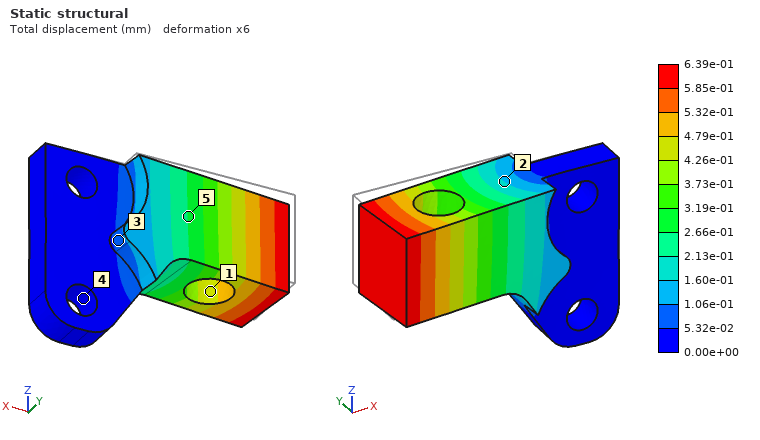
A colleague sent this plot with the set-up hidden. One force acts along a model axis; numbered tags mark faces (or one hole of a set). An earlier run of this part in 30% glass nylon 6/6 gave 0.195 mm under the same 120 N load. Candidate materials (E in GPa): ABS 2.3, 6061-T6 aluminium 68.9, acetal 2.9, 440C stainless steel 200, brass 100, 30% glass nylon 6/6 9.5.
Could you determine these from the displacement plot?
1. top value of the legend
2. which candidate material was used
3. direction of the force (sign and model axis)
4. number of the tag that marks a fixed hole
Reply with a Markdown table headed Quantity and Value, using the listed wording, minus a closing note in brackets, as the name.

| Quantity | Value |
|---|---|
| top value of the legend | 6.39e-01 mm |
| which candidate material was used | acetal |
| direction of the force | -Y |
| number of the tag that marks a fixed hole | 4 |
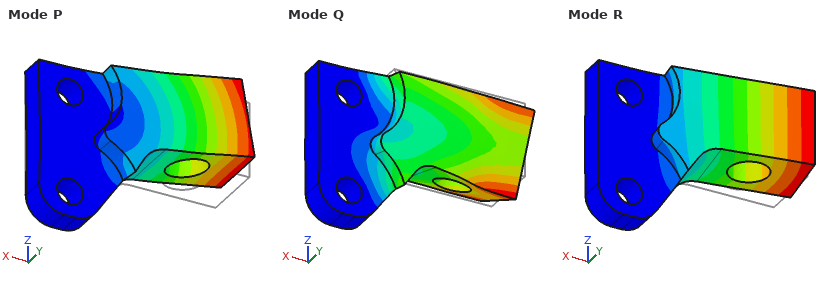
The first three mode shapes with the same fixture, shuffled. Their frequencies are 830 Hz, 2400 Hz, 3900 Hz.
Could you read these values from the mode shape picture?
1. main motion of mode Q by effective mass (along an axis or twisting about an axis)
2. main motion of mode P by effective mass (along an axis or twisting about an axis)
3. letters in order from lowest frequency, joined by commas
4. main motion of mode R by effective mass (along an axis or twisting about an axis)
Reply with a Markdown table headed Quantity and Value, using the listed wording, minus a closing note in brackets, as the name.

| Quantity | Value |
|---|---|
| main motion of mode Q by effective mass | twisting about X |
| main motion of mode P by effective mass | along Z |
| letters in order from lowest frequency, joined by commas | R, P, Q |
| main motion of mode R by effective mass | along Y |
